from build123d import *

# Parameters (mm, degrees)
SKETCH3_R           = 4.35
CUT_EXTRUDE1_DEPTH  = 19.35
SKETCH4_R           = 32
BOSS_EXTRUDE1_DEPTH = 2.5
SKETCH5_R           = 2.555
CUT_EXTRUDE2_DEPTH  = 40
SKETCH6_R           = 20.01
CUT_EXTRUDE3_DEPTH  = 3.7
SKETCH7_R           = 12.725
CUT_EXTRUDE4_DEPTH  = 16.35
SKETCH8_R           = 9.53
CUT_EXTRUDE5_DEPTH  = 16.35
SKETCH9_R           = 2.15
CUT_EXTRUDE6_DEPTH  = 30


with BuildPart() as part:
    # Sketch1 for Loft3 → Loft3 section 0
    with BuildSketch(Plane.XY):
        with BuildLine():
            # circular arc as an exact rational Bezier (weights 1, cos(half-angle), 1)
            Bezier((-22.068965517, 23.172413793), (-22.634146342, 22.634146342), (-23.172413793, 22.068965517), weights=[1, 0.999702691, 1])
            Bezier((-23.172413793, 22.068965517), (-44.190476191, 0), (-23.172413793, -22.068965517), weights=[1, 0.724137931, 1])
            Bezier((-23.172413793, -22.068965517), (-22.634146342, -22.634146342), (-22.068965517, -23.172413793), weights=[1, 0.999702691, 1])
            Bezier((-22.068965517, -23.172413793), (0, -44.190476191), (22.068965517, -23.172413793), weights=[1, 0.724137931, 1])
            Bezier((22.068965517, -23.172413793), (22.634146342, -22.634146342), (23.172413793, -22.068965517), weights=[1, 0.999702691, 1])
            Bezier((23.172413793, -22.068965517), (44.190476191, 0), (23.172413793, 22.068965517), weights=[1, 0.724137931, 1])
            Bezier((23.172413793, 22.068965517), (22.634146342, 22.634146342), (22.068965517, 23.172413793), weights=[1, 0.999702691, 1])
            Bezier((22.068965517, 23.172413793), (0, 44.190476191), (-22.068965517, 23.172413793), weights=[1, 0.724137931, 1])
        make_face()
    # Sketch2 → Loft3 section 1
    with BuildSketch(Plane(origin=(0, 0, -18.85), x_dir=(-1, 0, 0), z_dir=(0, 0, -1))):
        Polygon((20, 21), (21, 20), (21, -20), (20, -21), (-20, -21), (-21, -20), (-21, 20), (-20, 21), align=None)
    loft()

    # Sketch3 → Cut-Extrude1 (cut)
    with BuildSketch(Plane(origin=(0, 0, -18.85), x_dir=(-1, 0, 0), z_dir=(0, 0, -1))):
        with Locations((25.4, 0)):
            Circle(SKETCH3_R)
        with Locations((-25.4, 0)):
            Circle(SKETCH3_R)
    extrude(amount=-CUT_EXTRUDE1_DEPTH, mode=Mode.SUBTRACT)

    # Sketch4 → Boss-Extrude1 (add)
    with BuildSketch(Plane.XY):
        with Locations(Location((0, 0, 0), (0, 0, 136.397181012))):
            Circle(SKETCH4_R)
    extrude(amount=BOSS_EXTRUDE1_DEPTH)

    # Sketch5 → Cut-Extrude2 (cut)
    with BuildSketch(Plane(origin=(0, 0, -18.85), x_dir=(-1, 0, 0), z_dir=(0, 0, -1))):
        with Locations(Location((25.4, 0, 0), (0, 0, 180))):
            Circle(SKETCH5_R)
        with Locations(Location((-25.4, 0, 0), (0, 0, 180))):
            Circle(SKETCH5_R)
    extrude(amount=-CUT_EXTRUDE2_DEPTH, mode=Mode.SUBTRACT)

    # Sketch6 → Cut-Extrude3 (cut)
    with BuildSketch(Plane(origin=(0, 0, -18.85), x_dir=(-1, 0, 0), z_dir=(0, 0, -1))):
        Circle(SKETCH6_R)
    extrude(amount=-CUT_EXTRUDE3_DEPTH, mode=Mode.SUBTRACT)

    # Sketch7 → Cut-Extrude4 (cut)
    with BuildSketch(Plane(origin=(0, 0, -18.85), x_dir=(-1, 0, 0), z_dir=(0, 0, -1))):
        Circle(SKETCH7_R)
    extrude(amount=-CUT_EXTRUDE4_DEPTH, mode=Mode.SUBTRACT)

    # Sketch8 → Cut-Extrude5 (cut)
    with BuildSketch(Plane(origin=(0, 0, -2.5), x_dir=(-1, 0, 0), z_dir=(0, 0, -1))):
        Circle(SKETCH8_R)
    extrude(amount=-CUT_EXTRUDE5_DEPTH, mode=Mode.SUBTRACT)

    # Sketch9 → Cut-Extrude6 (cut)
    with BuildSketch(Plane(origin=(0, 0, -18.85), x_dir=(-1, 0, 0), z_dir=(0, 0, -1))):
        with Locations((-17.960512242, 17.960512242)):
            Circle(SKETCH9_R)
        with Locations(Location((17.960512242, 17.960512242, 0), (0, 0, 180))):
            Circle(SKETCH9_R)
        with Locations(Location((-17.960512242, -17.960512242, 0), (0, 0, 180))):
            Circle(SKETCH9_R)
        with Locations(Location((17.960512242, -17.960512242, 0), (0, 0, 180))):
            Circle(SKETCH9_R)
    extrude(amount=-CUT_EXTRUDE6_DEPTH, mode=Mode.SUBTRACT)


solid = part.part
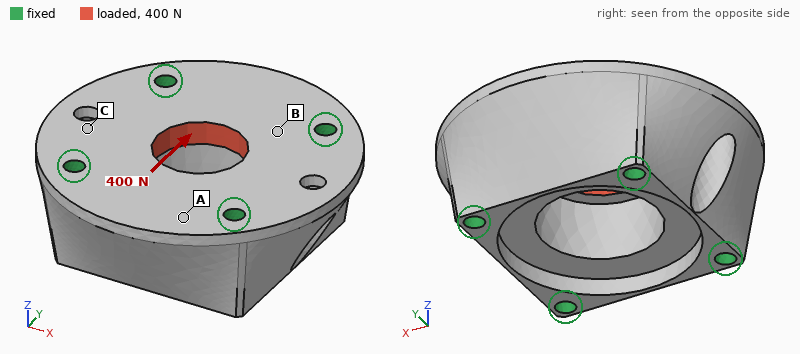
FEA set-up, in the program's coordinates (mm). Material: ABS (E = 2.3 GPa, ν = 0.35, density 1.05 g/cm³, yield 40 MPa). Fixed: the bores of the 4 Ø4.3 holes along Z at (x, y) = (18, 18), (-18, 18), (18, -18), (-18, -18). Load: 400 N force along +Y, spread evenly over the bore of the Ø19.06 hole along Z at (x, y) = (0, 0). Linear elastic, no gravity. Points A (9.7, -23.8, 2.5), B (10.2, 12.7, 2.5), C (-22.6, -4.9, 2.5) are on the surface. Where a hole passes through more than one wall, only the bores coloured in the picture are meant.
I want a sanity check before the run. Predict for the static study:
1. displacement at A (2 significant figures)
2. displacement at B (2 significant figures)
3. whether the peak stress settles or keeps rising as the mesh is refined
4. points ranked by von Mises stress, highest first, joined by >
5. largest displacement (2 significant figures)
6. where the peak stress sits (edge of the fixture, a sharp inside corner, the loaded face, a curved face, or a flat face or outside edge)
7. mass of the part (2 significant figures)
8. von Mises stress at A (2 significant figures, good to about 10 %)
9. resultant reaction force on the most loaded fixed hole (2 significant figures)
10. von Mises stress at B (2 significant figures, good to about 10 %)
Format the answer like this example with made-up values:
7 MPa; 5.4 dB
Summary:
4.9 µm; 5.2 µm; keeps rising; B > A > C; 13 µm; edge of the fixture; 41 g; 0.53 MPa; 100 N; 1.2 MPa
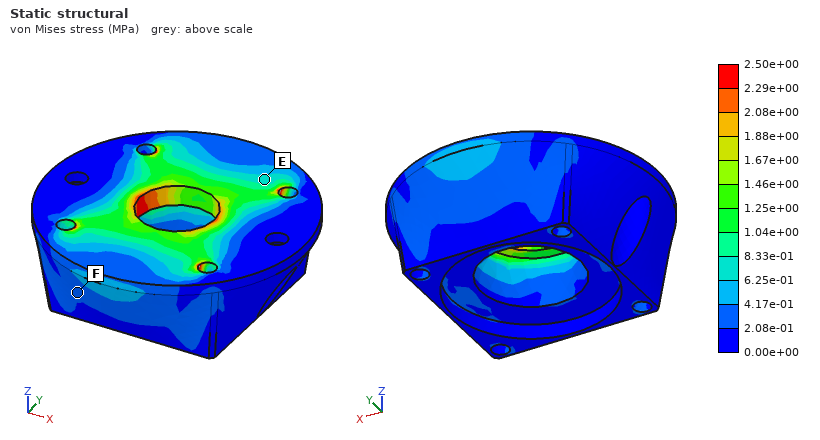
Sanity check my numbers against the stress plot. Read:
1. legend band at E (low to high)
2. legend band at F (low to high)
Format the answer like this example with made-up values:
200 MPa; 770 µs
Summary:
6.25e-01 to 8.33e-01 MPa; 2.08e-01 to 4.17e-01 MPa
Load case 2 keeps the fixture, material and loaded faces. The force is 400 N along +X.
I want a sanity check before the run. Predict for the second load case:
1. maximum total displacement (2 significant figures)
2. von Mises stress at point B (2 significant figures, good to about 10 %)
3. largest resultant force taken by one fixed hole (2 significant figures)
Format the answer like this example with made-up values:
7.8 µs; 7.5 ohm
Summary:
14 µm; 1.0 MPa; 110 N
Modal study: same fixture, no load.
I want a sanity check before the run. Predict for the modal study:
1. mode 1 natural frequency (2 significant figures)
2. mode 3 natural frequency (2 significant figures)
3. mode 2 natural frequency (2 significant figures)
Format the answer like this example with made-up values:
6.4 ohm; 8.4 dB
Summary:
8100 Hz; 9600 Hz; 9400 Hz
